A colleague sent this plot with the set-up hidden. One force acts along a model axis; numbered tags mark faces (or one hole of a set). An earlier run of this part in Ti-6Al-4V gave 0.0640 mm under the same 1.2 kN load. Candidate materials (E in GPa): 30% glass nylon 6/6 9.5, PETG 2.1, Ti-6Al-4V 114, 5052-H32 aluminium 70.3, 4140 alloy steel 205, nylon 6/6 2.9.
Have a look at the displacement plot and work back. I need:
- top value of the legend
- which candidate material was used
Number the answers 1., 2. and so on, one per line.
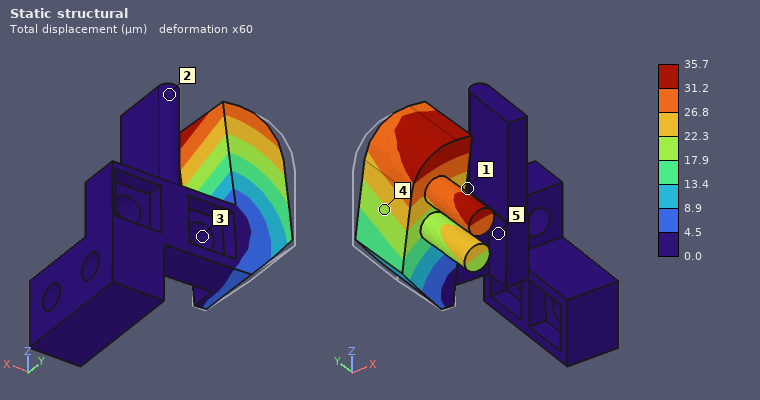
1. 35.7 µm
2. 4140 alloy steel
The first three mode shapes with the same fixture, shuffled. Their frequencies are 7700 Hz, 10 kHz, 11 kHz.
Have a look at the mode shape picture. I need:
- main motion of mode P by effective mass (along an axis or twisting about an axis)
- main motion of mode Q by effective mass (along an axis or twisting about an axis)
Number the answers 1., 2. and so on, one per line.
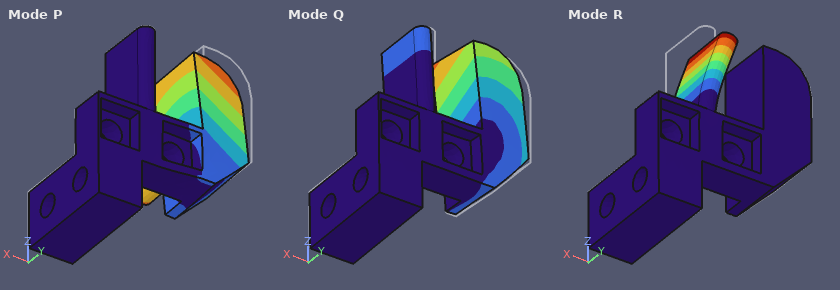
1. along Y
2. along X
